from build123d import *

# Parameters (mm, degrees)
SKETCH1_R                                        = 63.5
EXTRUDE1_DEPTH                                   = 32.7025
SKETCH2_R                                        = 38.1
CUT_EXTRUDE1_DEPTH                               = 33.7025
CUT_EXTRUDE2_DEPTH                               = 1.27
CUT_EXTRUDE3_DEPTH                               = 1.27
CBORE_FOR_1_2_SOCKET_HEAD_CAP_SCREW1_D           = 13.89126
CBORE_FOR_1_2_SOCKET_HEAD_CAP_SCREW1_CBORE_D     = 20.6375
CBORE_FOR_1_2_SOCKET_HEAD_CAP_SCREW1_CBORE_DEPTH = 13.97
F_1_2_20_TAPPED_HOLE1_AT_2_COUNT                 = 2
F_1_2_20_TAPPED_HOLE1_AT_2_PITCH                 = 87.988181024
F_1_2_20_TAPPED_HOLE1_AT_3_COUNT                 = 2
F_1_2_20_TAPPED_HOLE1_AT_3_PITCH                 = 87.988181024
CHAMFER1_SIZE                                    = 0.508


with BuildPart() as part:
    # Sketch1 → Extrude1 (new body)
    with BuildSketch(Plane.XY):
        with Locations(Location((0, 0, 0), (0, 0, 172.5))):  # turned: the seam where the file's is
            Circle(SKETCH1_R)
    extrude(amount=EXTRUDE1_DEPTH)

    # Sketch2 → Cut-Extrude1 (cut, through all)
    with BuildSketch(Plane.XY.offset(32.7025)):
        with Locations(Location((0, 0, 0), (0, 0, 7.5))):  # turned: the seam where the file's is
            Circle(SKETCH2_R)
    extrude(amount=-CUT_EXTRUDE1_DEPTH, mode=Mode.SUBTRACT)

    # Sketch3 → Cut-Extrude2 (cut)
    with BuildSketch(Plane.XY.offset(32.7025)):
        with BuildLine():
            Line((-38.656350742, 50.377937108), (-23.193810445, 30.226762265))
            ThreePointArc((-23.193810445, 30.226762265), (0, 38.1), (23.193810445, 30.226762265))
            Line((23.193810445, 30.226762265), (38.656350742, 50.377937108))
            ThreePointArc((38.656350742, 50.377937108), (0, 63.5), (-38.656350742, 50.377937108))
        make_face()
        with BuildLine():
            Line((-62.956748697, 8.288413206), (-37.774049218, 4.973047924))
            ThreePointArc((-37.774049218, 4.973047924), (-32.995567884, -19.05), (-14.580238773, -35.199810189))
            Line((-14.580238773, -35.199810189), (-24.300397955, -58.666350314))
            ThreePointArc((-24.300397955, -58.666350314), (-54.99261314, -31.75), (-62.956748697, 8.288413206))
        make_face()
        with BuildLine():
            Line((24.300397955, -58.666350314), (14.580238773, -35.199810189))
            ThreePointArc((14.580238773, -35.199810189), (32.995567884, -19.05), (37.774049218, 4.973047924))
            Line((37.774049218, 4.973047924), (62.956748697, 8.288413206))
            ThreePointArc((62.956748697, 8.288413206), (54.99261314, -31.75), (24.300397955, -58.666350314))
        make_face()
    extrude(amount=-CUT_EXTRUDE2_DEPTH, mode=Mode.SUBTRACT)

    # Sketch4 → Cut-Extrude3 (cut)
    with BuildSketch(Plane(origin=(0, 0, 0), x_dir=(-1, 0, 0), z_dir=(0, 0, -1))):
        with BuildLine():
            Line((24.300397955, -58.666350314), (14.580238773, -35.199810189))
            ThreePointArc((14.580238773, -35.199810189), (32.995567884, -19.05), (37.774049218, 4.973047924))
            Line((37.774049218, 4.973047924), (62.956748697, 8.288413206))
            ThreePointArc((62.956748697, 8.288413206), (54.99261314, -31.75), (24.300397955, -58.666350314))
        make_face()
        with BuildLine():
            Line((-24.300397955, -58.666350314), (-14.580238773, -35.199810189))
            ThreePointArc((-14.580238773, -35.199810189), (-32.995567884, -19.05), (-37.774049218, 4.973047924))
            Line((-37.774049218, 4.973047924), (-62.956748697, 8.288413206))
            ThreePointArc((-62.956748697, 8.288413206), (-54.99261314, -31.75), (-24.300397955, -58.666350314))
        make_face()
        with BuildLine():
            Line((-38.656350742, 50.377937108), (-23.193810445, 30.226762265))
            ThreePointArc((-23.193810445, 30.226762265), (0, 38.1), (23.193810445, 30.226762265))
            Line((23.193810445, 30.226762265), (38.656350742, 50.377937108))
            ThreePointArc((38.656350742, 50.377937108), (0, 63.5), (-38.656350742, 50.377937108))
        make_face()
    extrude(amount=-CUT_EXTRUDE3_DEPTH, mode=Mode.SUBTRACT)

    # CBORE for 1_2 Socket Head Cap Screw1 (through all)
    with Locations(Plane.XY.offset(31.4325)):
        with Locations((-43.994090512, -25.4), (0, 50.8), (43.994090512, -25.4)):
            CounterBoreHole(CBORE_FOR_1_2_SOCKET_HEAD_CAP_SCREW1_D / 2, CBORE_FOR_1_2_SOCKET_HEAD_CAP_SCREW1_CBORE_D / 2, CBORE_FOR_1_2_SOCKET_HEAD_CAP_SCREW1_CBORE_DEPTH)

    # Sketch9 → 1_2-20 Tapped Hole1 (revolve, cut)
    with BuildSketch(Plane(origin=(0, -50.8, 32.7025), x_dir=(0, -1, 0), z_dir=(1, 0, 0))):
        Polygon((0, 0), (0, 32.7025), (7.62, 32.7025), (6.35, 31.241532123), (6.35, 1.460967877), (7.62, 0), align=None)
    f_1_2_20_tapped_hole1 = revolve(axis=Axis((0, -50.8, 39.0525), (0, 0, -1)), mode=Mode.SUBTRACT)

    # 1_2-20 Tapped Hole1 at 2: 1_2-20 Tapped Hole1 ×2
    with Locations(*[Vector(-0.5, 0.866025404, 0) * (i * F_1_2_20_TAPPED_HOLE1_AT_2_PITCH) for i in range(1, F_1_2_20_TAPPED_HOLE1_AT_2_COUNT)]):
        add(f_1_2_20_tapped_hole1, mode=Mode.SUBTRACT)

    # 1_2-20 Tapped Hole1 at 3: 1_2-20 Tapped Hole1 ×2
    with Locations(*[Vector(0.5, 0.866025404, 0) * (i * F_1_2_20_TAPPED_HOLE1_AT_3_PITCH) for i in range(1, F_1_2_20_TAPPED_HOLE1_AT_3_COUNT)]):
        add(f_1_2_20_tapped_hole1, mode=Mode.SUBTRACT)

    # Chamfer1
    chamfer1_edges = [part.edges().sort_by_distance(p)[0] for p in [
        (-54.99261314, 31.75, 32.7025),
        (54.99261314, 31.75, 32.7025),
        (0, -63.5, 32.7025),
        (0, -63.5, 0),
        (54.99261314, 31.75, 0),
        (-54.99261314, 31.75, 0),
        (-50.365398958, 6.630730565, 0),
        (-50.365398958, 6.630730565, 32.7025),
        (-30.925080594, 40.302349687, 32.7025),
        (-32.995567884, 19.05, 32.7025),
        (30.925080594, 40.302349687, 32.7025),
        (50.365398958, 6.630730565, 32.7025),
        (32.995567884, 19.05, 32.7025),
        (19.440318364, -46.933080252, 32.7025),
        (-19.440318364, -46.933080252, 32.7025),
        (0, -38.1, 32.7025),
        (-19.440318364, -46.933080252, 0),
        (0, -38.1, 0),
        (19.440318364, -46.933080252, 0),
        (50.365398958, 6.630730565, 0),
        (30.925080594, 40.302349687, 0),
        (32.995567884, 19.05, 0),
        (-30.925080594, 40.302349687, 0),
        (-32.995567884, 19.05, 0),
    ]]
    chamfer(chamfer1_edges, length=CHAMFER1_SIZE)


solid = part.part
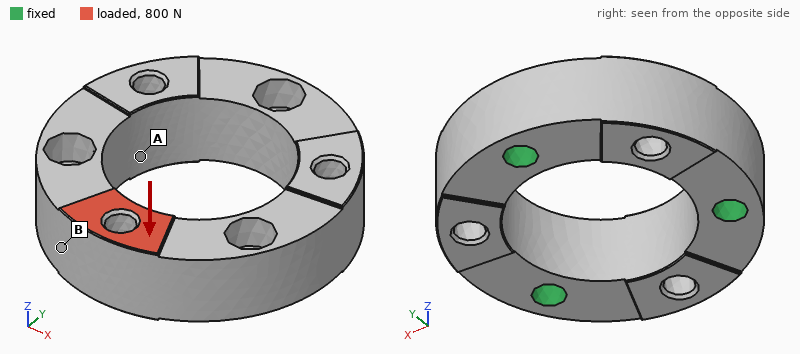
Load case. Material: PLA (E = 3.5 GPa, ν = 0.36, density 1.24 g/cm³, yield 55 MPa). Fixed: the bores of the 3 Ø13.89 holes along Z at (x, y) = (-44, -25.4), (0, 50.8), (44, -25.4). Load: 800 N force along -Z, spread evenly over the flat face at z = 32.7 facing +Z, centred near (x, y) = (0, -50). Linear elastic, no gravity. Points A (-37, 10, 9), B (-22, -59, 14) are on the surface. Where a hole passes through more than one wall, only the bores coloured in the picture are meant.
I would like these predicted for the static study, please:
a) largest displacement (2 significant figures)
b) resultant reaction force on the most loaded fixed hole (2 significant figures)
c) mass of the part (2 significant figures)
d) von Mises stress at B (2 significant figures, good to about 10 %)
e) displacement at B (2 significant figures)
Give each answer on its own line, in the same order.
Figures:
0.12 mm
440 N
270 g
1.7 MPa
0.077 mm
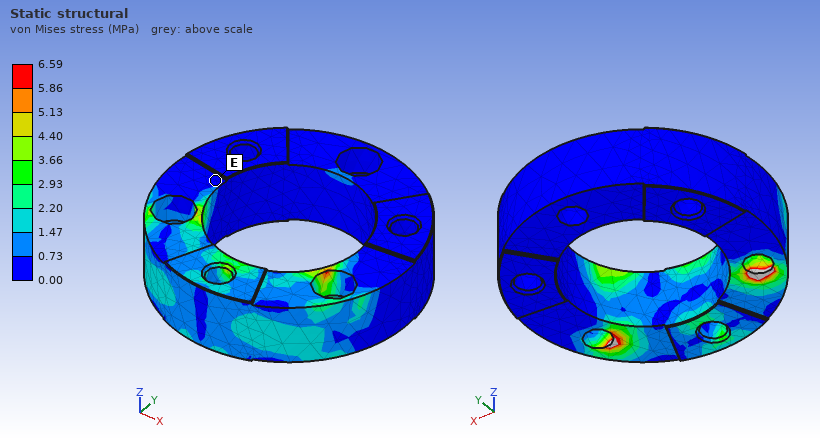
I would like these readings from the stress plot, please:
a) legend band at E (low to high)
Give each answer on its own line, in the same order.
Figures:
0.00 to 0.73 MPa
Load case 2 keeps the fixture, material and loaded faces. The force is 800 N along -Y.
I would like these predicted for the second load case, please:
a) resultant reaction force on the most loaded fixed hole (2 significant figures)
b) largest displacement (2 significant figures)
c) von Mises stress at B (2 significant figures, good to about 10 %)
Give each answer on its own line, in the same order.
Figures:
480 N
0.13 mm
1.9 MPa
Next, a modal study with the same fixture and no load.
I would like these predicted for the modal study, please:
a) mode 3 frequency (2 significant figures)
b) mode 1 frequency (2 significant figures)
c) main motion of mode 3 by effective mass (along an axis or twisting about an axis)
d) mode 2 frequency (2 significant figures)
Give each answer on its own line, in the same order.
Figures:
2500 Hz
2100 Hz
along Z
2100 Hz
